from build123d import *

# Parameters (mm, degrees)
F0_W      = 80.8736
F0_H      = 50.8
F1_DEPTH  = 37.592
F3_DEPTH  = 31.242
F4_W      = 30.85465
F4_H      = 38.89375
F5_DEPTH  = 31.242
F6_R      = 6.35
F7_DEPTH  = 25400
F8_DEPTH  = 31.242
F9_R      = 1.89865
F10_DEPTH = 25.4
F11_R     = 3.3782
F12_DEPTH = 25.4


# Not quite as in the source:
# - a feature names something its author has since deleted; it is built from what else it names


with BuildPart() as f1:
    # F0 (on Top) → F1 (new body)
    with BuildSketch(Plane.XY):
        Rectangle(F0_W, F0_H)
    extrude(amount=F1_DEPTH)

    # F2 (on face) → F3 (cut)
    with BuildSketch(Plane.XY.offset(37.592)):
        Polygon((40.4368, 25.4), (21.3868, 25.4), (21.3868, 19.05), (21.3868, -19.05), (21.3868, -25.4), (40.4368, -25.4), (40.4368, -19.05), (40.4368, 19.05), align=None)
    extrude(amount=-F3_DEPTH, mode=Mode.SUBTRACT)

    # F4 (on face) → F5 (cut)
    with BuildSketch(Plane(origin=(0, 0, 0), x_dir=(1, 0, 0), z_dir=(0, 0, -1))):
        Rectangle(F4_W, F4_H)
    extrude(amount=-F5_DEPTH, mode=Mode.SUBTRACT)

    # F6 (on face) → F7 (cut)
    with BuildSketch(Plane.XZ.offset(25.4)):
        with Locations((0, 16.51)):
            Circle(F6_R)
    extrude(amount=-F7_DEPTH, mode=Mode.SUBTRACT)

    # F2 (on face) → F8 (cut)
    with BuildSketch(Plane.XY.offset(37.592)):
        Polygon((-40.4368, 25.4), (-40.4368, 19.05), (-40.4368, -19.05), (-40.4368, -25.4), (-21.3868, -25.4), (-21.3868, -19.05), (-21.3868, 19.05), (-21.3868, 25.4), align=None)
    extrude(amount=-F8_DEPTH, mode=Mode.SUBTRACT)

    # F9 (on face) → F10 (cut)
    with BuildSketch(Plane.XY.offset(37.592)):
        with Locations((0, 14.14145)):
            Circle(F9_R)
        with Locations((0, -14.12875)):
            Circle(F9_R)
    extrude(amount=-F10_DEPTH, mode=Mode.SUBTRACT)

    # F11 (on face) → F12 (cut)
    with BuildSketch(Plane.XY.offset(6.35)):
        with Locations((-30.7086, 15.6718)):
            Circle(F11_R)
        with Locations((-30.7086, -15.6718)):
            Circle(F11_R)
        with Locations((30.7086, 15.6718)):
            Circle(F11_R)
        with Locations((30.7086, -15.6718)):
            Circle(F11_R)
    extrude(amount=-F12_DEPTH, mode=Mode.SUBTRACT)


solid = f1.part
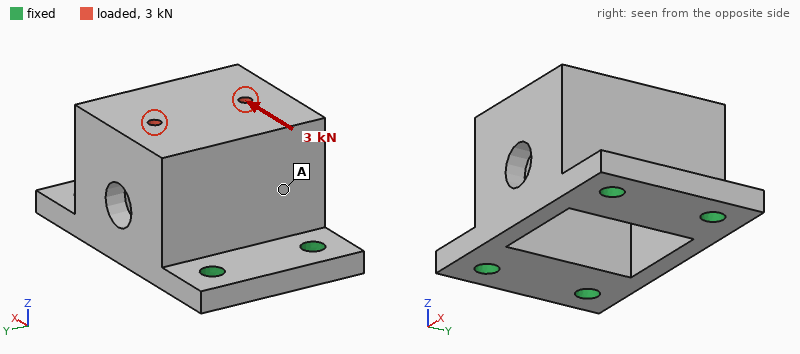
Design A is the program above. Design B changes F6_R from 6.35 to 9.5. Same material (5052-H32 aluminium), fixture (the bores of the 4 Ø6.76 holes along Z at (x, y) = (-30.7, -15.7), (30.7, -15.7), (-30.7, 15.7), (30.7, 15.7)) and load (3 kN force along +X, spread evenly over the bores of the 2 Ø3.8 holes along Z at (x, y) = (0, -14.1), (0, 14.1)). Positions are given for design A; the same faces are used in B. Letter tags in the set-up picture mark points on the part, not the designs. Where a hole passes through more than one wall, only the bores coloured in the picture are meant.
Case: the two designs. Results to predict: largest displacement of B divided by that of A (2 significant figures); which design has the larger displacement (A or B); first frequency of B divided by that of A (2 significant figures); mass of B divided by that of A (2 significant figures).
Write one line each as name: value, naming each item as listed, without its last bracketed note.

largest displacement of B divided by that of A: 1.2
which design has the larger displacement: B
first frequency of B divided by that of A: 1.0
mass of B divided by that of A: 0.97
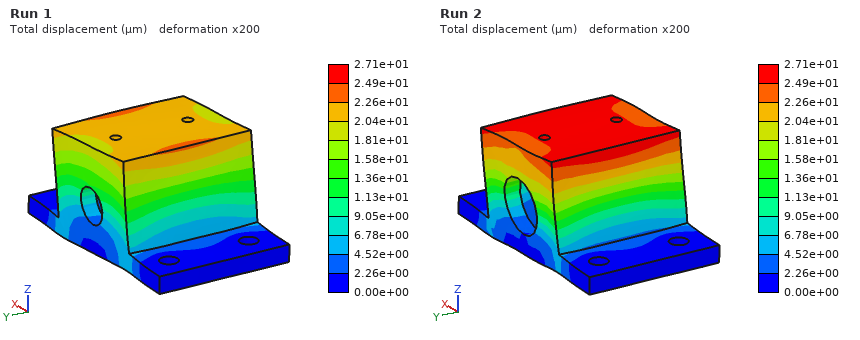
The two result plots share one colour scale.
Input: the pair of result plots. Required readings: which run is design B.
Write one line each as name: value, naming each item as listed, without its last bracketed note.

which run is design B: Run 2
